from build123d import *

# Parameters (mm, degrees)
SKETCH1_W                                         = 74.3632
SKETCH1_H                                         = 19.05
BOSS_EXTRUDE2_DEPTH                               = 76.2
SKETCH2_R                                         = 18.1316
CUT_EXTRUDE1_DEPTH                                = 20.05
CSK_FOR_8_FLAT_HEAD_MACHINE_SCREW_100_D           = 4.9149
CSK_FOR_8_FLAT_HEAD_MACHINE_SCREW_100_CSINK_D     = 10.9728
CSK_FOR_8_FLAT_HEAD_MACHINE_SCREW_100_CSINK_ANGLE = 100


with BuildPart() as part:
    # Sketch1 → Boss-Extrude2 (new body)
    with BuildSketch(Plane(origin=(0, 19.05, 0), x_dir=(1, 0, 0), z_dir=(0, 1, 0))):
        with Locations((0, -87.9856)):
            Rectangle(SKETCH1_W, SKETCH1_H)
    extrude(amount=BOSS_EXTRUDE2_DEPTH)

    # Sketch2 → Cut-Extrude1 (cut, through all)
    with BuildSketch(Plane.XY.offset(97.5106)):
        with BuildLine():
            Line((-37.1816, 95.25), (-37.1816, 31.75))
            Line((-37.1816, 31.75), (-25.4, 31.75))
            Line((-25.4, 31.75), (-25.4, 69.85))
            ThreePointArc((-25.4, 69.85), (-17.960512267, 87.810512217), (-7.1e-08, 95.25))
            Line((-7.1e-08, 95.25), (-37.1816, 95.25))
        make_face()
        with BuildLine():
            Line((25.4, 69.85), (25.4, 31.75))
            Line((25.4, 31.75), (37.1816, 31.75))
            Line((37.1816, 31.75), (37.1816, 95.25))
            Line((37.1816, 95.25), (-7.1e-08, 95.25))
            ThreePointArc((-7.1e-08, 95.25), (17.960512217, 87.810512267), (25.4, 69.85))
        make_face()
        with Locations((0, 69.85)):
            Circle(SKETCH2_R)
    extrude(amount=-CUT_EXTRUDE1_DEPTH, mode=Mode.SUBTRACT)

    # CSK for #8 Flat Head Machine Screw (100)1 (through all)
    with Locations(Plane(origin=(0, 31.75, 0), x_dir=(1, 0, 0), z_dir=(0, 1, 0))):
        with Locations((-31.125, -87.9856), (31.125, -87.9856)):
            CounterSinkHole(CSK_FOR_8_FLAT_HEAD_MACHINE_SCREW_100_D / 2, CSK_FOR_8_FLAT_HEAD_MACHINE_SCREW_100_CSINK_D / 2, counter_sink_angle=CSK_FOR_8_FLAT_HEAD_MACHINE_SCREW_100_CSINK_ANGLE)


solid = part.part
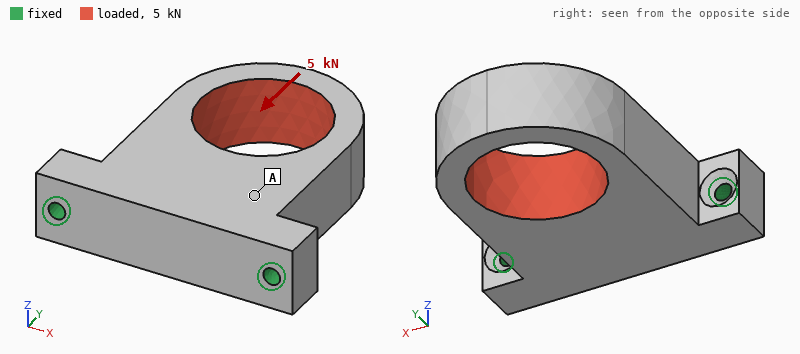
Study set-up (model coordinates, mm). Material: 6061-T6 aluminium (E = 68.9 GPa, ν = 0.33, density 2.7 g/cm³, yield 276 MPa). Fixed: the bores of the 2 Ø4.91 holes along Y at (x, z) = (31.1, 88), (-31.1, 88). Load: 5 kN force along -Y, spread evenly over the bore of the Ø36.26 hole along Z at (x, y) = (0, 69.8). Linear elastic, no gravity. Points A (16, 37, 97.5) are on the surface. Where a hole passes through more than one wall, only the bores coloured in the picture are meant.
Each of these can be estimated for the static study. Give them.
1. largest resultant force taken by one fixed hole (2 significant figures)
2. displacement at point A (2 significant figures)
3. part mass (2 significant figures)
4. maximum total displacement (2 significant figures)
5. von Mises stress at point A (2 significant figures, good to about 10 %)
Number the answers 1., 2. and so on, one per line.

1. 2.7 kN
2. 8.0 µm
3. 150 g
4. 25 µm
5. 6.5 MPa
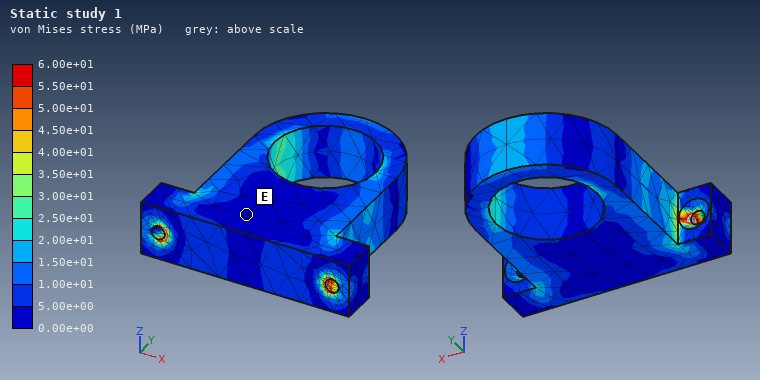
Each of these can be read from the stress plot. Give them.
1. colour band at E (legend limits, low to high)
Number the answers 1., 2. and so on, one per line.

1. 0.00e+00 to 5.00e+00 MPa
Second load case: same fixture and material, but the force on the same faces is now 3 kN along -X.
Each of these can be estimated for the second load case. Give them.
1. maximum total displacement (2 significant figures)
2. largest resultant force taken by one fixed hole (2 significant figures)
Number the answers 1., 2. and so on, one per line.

1. 73 µm
2. 2.8 kN
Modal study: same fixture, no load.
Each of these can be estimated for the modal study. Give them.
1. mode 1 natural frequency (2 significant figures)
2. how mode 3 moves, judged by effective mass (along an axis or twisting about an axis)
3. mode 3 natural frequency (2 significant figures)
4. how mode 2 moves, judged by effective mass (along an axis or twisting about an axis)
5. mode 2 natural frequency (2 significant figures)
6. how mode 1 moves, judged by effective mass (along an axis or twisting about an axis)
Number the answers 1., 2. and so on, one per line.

1. 2100 Hz
2. twisting about Y
3. 7100 Hz
4. along X
5. 5000 Hz
6. along Z
